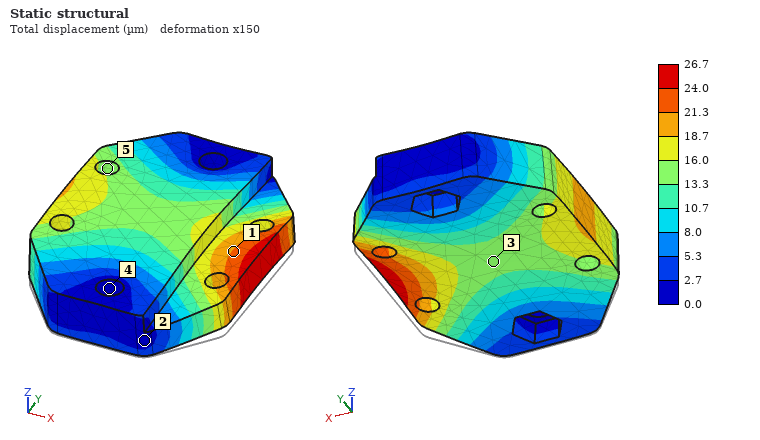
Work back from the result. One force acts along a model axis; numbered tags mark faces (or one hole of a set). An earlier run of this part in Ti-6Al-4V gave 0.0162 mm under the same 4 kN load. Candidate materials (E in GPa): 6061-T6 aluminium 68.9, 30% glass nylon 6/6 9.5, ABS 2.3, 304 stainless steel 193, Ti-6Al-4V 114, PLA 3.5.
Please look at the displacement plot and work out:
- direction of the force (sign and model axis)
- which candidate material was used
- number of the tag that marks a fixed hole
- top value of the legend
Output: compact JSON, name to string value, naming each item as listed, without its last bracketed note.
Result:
{"direction of the force": "+Z", "which candidate material was used": "6061-T6 aluminium", "number of the tag that marks a fixed hole": "4", "top value of the legend": "26.7 µm"}
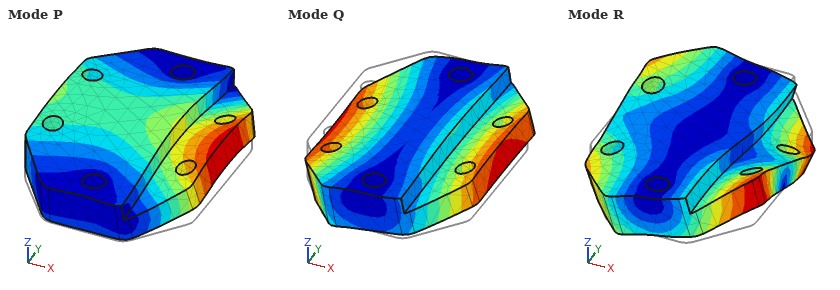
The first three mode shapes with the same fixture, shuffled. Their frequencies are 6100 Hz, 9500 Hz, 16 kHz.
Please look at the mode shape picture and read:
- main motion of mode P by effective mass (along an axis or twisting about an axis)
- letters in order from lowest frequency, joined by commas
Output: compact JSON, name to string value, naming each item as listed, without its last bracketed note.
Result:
{"main motion of mode P by effective mass": "along Z", "letters in order from lowest frequency, joined by commas": "Q, P, R"}
